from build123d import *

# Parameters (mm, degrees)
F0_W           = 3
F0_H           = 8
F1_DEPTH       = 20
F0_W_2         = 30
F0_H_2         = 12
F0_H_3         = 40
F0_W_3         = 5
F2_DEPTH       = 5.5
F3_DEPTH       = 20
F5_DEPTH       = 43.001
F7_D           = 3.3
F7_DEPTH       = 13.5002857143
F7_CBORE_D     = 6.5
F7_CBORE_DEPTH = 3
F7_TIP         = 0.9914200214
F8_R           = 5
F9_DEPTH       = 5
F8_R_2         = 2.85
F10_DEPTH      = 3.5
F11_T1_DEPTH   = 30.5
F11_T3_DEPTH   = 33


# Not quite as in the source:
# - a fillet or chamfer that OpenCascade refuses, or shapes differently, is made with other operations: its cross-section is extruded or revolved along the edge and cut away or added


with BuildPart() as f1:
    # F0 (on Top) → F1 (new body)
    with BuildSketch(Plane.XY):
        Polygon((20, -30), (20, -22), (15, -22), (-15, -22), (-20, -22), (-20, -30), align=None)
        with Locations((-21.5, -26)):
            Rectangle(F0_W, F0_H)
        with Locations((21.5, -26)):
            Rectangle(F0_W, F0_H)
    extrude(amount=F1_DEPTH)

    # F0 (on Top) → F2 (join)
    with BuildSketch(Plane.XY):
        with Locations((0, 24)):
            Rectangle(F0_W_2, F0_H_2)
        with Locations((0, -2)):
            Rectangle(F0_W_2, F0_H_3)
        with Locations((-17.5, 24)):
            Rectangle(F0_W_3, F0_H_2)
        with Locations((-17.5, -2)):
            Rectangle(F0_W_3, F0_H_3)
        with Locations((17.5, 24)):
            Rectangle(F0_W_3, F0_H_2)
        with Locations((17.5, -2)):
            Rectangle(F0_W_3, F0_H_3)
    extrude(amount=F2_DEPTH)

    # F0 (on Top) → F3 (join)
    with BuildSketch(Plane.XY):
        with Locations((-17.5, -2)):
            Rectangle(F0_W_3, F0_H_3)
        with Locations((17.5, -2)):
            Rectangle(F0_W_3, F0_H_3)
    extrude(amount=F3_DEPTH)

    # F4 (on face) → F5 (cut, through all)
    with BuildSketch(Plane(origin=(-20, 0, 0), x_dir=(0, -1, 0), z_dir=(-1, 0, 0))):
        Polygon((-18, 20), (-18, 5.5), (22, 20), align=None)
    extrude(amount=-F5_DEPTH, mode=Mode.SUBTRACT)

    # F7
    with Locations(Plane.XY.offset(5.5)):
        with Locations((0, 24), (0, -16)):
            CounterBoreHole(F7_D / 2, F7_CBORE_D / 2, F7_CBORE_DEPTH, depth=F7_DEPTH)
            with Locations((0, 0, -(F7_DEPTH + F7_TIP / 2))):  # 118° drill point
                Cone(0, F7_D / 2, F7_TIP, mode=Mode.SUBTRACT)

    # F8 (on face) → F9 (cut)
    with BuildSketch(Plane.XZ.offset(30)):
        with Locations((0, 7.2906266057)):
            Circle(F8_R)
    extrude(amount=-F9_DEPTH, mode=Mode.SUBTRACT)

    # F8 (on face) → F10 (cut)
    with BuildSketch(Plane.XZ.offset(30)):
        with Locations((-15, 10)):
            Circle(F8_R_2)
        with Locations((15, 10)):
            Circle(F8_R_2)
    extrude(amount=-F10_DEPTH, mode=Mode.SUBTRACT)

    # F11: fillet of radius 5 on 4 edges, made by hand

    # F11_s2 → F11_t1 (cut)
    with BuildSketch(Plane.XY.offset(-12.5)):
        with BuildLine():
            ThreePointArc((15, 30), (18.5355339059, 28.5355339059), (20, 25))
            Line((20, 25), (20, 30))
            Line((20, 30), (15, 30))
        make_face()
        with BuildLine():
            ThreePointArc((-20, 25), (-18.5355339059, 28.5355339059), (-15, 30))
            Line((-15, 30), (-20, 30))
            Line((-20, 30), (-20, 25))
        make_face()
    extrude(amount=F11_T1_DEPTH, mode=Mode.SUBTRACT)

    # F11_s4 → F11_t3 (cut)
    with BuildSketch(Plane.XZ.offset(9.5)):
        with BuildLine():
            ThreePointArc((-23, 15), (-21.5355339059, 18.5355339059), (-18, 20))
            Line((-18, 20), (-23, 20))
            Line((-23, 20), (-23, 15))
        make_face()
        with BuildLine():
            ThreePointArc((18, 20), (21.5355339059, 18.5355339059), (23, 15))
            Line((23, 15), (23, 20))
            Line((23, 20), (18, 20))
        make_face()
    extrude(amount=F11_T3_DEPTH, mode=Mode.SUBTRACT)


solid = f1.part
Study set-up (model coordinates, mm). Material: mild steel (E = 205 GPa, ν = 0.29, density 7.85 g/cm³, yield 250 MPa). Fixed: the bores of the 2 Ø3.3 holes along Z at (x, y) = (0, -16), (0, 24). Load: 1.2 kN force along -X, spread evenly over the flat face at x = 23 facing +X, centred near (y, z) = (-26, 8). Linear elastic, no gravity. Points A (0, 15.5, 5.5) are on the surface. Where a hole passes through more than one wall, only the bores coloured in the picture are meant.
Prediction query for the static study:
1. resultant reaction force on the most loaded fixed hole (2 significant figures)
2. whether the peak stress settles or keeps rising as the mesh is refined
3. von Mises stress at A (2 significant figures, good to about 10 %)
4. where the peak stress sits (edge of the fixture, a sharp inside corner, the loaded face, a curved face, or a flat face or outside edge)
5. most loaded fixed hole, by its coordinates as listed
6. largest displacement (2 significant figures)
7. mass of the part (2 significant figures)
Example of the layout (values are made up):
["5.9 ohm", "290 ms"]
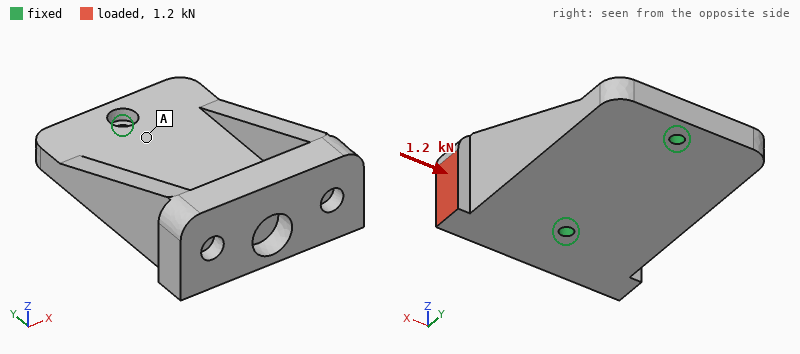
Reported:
["1.5 kN", "keeps rising", "17 MPa", "edge of the fixture", "(0, -16)", "40 µm", "160 g"]
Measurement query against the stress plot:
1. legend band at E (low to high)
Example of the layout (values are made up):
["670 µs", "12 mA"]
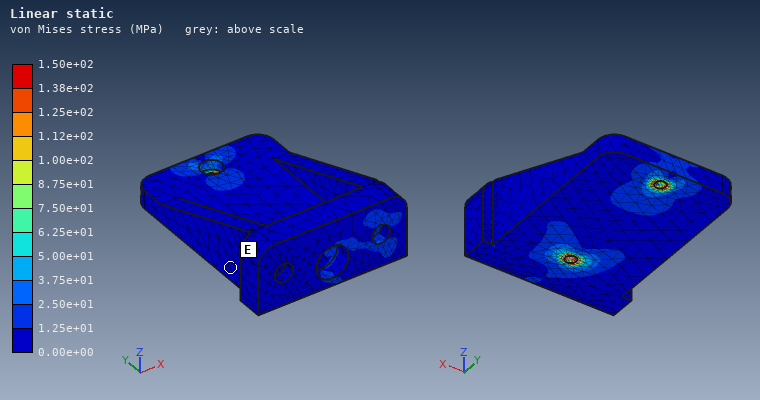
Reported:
["0.00e+00 to 1.25e+01 MPa"]
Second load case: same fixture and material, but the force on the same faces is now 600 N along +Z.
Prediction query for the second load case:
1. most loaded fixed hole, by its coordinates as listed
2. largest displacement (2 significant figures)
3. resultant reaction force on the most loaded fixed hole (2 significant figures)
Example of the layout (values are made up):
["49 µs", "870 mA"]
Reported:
["(0, -16)", "76 µm", "760 N"]
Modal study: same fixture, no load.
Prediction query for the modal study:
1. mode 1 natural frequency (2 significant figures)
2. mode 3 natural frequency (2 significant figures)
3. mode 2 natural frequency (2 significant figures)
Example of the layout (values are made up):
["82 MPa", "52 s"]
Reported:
["2100 Hz", "7500 Hz", "6300 Hz"]
